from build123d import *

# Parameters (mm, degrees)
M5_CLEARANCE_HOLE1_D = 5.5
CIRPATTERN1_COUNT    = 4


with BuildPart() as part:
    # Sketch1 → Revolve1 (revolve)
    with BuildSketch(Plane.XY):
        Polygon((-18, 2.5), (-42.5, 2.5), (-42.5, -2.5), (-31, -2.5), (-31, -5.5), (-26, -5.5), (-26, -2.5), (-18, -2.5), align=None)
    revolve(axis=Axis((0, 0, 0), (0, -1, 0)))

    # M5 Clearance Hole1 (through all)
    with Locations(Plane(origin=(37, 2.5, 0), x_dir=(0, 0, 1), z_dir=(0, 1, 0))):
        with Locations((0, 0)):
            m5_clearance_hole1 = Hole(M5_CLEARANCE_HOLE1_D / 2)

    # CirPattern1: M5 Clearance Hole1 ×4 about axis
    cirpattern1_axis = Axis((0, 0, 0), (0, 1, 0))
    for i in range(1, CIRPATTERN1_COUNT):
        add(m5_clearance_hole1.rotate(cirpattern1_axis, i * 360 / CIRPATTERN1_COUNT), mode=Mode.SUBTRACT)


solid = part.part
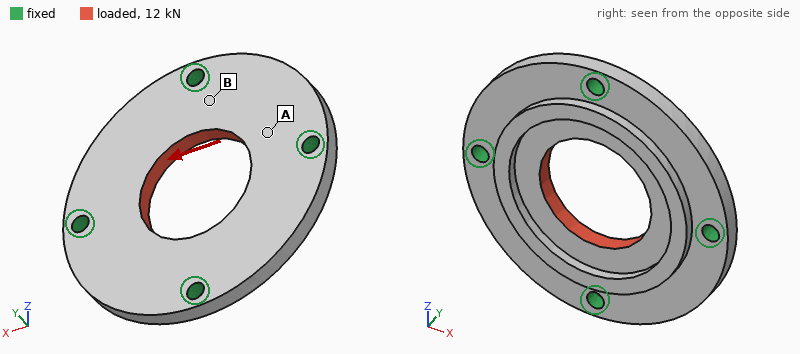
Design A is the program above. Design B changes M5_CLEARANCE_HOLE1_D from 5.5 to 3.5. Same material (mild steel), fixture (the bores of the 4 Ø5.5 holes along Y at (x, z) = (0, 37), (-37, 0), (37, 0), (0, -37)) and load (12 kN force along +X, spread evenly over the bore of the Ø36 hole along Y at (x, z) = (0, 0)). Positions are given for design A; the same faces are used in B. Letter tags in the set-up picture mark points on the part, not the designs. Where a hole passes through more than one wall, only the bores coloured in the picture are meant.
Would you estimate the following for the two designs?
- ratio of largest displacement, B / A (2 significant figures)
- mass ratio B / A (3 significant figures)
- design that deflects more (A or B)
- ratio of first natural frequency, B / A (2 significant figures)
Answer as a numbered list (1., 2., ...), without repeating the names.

1. 1.1
2. 1.01
3. B
4. 0.88
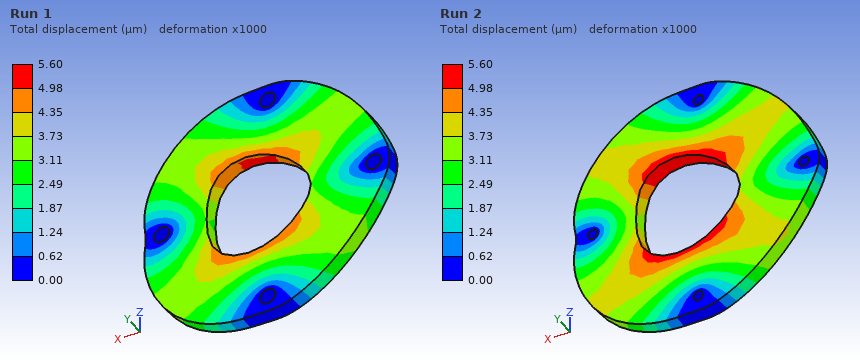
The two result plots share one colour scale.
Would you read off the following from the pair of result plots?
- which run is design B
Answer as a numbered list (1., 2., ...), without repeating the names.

1. Run 2
